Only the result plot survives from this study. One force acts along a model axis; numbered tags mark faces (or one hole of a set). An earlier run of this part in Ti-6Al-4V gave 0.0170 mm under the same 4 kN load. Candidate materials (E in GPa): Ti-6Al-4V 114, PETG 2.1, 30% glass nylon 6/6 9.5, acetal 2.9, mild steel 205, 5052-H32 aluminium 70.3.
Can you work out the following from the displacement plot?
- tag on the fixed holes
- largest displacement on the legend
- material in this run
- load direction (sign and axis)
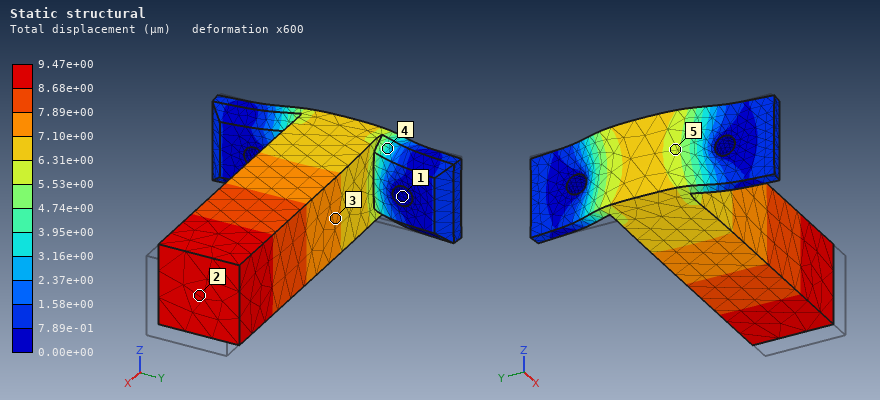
1
9.47e+00 µm
mild steel
-X
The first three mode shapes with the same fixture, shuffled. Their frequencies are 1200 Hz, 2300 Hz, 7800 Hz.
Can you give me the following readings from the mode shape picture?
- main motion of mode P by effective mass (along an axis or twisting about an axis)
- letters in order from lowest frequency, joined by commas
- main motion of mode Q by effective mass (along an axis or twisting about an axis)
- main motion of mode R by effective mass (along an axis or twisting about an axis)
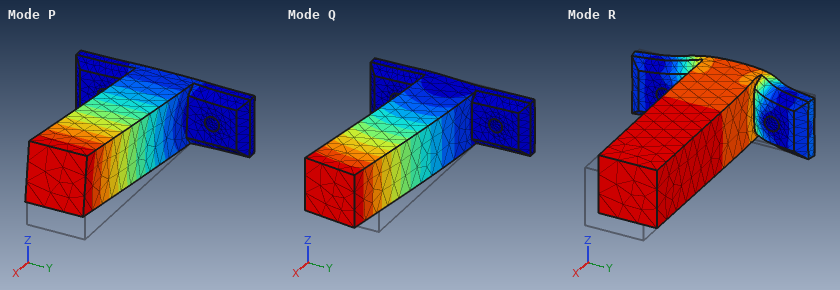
along Z
P, Q, R
along Y
along X
